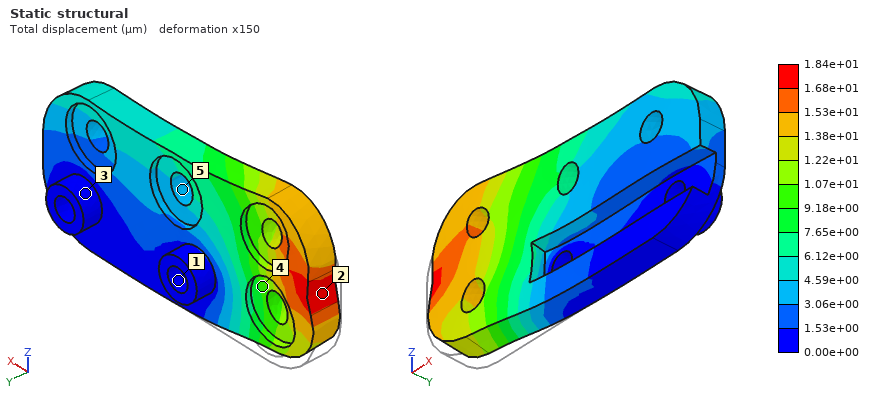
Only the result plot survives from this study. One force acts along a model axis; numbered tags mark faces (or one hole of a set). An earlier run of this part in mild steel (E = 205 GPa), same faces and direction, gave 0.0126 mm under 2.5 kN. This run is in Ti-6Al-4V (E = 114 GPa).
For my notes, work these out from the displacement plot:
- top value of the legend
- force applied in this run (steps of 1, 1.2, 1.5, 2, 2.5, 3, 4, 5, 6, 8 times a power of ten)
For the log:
1.84e+01 µm
2 kN
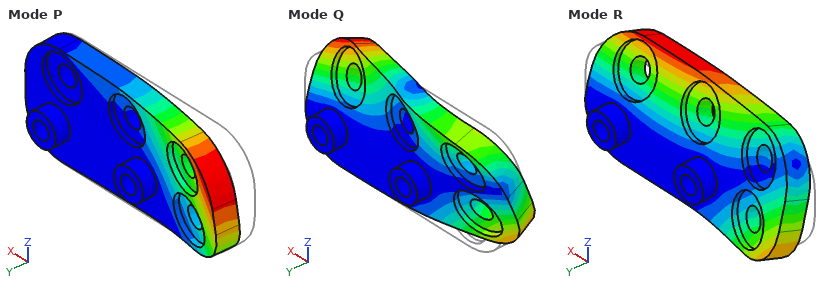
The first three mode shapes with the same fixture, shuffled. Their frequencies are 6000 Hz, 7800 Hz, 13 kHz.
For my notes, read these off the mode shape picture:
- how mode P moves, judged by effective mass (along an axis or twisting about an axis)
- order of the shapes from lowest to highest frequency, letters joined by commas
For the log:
along Y
P, R, Q
